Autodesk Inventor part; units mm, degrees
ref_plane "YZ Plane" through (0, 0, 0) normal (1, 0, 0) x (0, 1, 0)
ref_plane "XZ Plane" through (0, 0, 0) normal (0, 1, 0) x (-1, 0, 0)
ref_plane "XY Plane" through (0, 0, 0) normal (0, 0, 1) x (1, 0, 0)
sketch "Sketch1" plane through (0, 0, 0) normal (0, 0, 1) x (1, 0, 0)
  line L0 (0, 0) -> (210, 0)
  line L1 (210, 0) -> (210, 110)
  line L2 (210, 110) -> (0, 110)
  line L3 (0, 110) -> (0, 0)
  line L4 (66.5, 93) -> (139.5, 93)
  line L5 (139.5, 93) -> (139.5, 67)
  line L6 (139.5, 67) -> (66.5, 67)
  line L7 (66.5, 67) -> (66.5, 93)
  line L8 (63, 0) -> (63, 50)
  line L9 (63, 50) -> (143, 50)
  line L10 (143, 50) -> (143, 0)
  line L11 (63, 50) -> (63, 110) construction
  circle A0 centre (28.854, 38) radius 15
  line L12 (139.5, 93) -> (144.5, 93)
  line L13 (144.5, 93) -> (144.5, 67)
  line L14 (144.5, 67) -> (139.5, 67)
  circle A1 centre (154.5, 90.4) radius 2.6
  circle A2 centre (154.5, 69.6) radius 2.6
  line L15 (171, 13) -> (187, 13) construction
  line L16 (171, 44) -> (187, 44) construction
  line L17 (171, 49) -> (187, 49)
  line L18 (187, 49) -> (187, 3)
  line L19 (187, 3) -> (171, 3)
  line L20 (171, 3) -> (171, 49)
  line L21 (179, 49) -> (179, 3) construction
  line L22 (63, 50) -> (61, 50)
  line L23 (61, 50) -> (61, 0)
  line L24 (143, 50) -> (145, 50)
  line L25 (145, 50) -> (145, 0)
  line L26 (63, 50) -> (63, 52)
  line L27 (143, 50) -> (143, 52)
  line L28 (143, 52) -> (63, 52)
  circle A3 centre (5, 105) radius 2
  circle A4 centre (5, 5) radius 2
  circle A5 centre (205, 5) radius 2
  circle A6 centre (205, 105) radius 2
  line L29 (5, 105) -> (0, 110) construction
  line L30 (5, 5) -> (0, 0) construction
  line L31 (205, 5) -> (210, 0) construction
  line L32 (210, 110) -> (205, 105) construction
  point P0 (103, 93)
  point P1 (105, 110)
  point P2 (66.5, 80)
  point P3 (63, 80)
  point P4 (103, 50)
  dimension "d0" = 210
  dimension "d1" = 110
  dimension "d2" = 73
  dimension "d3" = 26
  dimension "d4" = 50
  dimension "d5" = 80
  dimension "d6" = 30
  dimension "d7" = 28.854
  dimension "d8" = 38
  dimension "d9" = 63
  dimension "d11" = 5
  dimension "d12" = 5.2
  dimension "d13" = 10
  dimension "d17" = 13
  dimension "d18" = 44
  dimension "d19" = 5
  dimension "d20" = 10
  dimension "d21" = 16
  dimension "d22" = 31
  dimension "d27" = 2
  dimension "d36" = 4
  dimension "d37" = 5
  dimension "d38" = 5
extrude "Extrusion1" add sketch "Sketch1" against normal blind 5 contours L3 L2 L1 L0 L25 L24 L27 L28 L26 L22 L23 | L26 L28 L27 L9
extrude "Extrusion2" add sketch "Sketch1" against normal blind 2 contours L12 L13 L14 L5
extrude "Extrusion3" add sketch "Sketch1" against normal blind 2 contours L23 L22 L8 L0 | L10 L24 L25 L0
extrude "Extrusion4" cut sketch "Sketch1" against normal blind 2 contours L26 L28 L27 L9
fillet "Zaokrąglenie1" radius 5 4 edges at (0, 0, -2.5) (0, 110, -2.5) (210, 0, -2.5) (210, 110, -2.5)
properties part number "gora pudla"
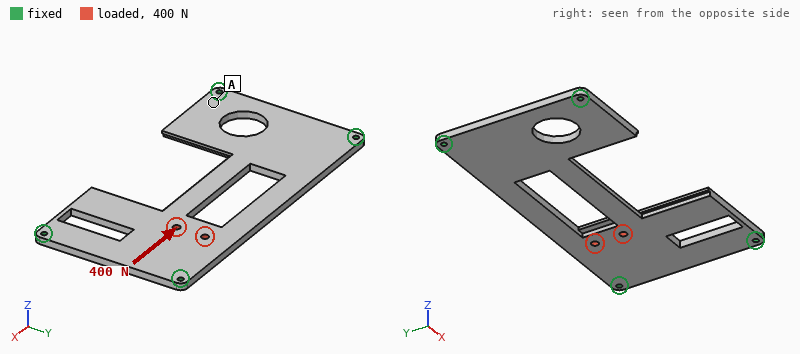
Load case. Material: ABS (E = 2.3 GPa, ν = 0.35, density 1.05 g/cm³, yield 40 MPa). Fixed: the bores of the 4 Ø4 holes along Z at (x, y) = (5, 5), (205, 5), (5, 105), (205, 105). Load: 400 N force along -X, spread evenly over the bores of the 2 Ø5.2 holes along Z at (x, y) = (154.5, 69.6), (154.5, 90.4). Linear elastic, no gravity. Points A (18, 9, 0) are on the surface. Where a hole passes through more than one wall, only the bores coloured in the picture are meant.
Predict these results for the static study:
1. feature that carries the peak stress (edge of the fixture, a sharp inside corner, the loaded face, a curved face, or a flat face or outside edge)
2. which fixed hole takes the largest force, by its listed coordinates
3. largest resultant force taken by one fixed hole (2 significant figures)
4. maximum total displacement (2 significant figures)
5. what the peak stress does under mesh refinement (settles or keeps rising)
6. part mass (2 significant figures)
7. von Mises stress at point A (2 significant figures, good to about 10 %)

edge of the fixture
(205, 105)
230 N
82 µm
keeps rising
81 g
0.43 MPa
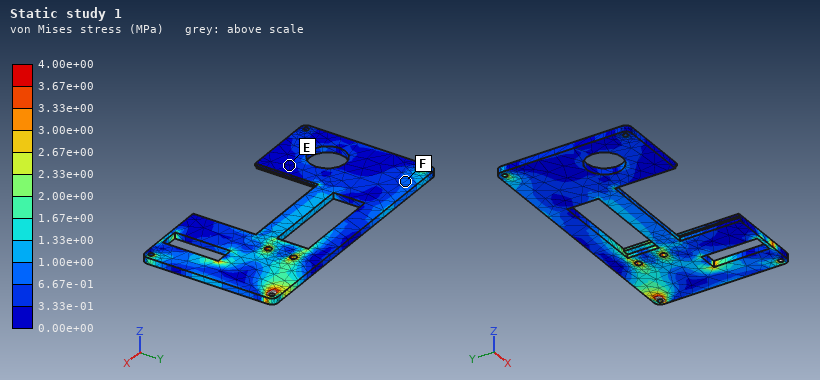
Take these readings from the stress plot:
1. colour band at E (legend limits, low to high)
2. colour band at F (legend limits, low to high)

0.00e+00 to 3.33e-01 MPa
6.67e-01 to 1.00e+00 MPa
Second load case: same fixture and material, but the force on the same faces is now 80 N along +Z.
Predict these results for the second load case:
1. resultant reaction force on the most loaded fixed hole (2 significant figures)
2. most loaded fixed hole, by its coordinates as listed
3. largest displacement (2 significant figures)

51 N
(205, 105)
2.4 mm
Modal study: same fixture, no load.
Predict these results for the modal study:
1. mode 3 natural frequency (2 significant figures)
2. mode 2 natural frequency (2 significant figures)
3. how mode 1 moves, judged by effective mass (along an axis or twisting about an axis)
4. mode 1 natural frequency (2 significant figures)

350 Hz
330 Hz
along Z
160 Hz
